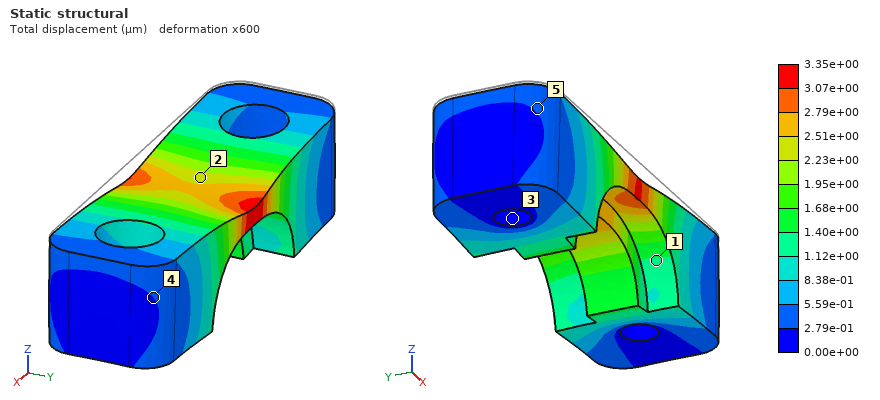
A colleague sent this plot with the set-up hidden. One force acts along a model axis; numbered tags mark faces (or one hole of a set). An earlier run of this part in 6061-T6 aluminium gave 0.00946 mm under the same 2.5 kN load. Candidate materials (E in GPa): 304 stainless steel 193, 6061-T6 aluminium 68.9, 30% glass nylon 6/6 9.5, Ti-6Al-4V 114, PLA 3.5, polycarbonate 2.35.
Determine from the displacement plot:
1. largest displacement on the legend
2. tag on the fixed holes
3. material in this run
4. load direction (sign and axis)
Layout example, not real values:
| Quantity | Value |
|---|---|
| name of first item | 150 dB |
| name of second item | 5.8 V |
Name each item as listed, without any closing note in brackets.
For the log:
| Quantity | Value |
|---|---|
| largest displacement on the legend | 3.35e+00 µm |
| tag on the fixed holes | 3 |
| material in this run | 304 stainless steel |
| load direction | -Z |
